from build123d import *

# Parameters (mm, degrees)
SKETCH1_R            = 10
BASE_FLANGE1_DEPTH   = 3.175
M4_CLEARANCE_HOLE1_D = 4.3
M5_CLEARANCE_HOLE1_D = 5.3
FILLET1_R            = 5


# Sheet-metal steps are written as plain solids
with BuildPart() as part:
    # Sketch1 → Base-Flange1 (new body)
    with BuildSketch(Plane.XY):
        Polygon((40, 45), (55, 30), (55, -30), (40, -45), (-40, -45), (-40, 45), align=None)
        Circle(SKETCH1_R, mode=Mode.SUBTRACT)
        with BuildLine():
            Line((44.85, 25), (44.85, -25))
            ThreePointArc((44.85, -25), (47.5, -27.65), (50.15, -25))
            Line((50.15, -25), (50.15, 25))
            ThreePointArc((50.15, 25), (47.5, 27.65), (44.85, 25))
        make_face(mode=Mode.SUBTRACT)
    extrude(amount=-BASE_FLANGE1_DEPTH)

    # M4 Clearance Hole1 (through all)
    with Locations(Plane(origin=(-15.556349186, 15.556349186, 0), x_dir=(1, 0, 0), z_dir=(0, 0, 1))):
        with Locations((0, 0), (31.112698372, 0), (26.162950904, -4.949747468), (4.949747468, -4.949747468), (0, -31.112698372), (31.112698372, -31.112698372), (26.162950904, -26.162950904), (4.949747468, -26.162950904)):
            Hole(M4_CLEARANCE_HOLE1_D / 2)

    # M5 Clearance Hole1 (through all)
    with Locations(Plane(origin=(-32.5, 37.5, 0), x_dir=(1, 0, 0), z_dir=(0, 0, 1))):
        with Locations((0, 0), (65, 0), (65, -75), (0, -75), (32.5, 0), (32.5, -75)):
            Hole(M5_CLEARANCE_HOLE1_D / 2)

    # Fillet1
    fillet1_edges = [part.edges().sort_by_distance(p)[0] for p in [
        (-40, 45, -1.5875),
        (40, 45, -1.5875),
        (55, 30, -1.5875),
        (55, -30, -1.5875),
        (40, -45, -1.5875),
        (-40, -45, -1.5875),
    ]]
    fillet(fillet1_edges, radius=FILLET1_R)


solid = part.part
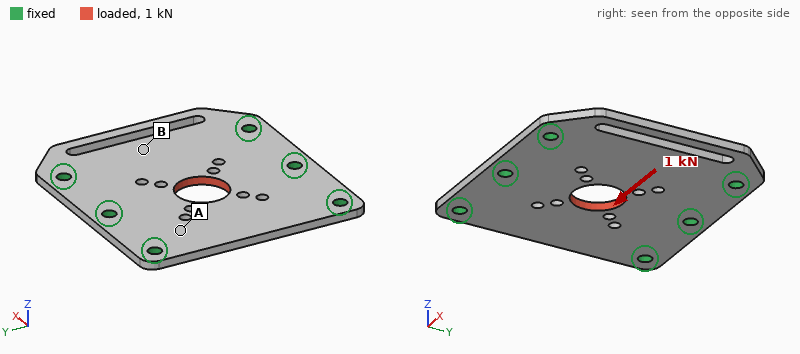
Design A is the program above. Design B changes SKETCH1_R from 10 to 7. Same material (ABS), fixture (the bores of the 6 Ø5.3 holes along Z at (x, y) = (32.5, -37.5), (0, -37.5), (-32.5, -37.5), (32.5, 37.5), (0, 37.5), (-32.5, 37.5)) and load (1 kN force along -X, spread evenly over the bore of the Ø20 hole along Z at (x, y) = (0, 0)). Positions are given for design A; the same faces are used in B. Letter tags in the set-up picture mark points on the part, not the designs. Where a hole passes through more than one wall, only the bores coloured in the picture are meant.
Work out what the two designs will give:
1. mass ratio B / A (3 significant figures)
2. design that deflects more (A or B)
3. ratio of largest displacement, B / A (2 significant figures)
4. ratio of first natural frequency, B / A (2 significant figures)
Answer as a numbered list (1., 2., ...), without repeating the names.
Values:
1. 1.02
2. B
3. 1.1
4. 1.00
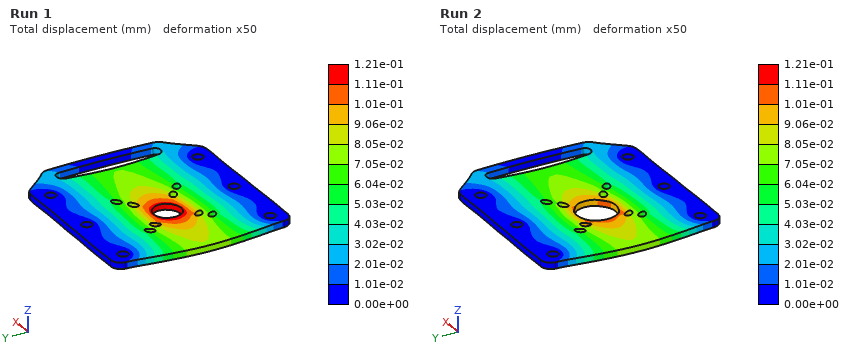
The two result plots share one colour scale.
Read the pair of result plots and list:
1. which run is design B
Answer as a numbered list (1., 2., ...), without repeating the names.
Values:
1. Run 1
